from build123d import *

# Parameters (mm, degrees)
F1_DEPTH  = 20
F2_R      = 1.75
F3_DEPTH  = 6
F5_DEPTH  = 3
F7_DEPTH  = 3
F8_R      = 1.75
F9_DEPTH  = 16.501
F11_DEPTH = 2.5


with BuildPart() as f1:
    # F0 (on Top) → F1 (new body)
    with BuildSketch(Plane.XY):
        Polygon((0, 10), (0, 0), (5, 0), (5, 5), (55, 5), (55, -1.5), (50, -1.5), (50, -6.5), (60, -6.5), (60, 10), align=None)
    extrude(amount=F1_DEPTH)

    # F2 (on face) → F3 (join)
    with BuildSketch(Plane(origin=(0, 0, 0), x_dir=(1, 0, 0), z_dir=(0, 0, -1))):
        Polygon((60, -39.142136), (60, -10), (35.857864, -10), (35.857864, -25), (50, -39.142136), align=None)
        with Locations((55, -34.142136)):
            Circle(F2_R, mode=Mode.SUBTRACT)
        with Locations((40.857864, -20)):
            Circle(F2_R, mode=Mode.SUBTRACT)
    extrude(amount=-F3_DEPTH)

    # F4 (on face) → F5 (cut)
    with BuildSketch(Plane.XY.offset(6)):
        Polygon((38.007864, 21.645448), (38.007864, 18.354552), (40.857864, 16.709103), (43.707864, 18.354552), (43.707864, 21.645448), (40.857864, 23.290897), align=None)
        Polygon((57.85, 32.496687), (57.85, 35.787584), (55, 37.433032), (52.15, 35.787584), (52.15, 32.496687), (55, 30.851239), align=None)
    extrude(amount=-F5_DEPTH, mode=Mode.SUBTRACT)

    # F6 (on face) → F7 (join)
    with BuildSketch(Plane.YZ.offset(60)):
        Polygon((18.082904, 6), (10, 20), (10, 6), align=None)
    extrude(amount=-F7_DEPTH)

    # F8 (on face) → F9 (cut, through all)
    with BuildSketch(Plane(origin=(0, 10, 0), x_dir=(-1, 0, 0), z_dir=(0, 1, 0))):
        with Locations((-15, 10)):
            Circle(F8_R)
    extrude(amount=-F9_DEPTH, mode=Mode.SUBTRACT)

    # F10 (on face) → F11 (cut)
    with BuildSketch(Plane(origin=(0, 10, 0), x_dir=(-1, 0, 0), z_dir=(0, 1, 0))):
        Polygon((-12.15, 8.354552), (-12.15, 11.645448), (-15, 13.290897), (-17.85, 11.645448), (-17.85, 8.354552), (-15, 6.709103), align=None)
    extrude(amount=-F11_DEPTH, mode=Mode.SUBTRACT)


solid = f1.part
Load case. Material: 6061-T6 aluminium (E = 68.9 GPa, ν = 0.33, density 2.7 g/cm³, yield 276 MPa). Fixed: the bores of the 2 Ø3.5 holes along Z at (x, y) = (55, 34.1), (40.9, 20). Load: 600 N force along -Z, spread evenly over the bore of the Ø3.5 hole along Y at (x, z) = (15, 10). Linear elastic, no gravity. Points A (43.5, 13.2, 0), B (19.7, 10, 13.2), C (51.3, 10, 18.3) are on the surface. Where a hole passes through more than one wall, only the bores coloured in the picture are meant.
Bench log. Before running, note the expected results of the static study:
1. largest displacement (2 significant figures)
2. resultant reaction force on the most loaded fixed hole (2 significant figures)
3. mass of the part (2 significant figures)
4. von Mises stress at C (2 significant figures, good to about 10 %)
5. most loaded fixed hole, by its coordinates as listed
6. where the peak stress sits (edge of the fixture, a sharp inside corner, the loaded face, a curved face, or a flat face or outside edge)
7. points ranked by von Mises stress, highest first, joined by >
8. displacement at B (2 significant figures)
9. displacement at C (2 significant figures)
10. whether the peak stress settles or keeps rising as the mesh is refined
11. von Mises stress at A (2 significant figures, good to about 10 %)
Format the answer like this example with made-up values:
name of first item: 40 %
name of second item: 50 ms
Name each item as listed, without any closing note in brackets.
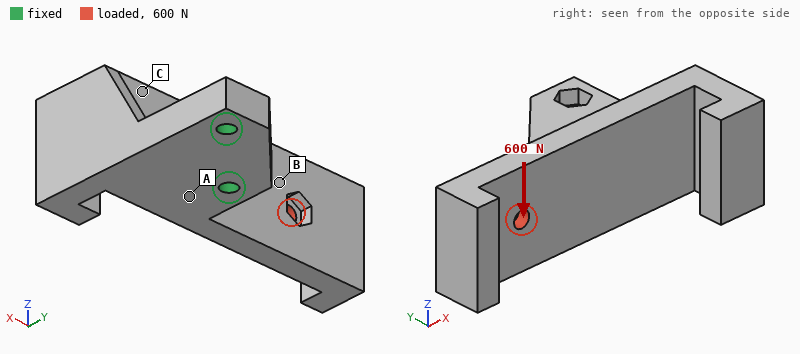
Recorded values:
largest displacement: 0.41 mm
resultant reaction force on the most loaded fixed hole: 1.4 kN
mass of the part: 31 g
von Mises stress at C: 38 MPa
most loaded fixed hole, by its coordinates as listed: (40.9, 20)
where the peak stress sits: edge of the fixture
points ranked by von Mises stress, highest first, joined by >: A > C > B
displacement at B: 0.21 mm
displacement at C: 0.11 mm
whether the peak stress settles or keeps rising as the mesh is refined: keeps rising
von Mises stress at A: 100 MPa
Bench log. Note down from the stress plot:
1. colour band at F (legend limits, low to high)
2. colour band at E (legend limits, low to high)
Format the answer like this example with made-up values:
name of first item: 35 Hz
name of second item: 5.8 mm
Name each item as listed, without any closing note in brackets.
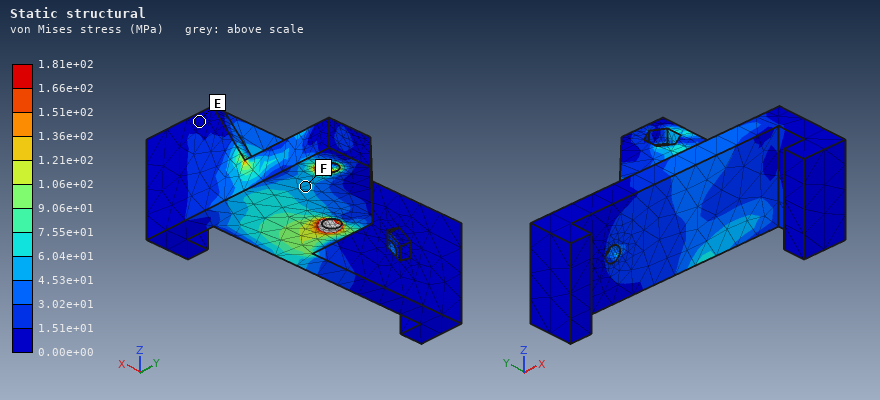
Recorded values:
colour band at F: 4.53e+01 to 6.04e+01 MPa
colour band at E: 0.00e+00 to 1.51e+01 MPa
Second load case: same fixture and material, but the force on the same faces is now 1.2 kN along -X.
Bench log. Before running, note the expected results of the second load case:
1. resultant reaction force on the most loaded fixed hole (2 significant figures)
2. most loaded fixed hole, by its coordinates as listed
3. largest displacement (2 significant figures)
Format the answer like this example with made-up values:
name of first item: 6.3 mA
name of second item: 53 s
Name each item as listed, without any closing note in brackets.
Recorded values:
resultant reaction force on the most loaded fixed hole: 1.6 kN
most loaded fixed hole, by its coordinates as listed: (40.9, 20)
largest displacement: 0.21 mm
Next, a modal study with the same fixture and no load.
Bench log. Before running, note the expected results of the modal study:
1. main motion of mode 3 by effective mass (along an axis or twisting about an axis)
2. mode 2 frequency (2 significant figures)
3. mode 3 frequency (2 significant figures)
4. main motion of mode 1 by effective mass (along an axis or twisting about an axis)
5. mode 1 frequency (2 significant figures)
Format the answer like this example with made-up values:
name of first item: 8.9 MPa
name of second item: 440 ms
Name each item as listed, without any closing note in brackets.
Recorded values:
main motion of mode 3 by effective mass: along Z
mode 2 frequency: 2000 Hz
mode 3 frequency: 3000 Hz
main motion of mode 1 by effective mass: along Y
mode 1 frequency: 1800 Hz
